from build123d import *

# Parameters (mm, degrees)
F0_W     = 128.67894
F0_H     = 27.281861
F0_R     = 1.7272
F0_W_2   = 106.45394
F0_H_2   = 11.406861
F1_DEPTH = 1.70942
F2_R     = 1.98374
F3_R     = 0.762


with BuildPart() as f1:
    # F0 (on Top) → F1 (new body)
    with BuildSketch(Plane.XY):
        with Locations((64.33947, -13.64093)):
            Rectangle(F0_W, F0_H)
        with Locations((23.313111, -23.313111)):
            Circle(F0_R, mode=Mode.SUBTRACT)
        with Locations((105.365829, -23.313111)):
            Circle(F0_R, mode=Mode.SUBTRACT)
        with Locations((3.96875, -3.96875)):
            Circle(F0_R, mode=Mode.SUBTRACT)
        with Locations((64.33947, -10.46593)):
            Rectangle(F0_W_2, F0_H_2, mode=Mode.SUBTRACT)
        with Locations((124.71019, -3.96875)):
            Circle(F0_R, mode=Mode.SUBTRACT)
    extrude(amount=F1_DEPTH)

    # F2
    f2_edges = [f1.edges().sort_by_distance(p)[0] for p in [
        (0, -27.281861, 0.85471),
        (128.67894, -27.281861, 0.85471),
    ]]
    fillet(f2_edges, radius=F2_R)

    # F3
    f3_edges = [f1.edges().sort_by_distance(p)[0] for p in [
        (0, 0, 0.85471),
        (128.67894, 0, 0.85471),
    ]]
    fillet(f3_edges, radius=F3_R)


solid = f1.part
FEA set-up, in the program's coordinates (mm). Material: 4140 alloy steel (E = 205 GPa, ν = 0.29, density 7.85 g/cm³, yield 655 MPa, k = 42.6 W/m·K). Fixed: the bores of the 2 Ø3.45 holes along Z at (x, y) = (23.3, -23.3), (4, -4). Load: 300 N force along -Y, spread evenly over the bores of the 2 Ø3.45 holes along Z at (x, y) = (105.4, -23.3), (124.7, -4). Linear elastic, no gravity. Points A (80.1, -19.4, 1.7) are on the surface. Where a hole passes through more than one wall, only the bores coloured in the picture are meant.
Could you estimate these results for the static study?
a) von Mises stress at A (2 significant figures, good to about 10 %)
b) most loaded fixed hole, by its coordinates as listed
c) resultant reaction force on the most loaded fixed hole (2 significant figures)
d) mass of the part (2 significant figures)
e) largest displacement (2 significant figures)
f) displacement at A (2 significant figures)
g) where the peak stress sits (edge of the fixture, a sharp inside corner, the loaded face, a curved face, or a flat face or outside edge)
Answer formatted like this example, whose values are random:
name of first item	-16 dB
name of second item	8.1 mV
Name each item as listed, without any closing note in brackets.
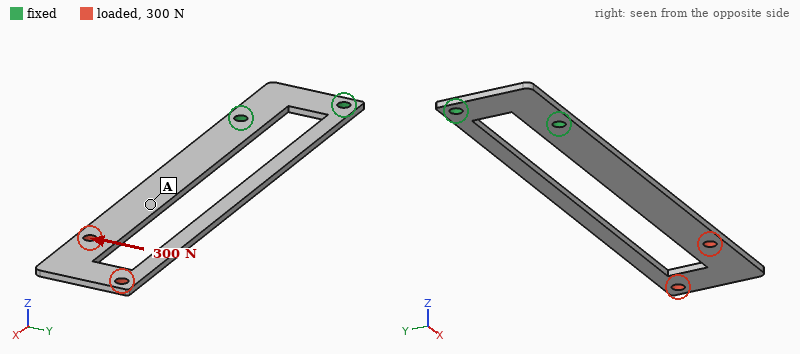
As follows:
von Mises stress at A	56 MPa
most loaded fixed hole, by its coordinates as listed	(23.3, -23.3)
resultant reaction force on the most loaded fixed hole	920 N
mass of the part	30 g
largest displacement	0.84 mm
displacement at A	0.46 mm
where the peak stress sits	edge of the fixture
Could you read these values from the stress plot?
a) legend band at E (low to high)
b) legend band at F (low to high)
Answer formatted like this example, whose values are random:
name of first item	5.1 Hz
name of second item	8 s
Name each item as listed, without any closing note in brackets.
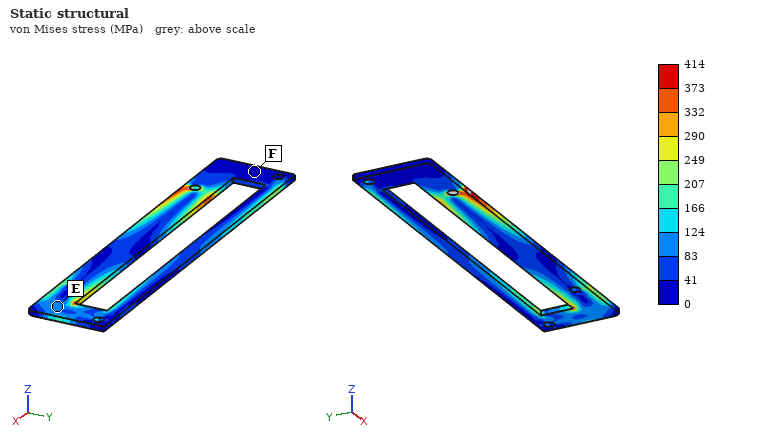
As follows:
legend band at E	83 to 124 MPa
legend band at F	0 to 41 MPa
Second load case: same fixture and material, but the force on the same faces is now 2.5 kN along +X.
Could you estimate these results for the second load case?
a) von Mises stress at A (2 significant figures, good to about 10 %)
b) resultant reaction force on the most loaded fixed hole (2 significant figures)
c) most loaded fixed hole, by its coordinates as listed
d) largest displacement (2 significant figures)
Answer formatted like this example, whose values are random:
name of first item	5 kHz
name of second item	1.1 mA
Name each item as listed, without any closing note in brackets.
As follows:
von Mises stress at A	82 MPa
resultant reaction force on the most loaded fixed hole	1.4 kN
most loaded fixed hole, by its coordinates as listed	(23.3, -23.3)
largest displacement	0.12 mm
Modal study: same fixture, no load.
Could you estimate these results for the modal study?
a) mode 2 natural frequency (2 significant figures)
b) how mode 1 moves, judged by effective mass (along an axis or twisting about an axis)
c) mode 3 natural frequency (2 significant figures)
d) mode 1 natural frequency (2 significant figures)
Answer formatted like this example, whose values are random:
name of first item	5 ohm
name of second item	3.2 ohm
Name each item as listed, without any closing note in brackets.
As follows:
mode 2 natural frequency	550 Hz
how mode 1 moves, judged by effective mass	along Z
mode 3 natural frequency	710 Hz
mode 1 natural frequency	110 Hz
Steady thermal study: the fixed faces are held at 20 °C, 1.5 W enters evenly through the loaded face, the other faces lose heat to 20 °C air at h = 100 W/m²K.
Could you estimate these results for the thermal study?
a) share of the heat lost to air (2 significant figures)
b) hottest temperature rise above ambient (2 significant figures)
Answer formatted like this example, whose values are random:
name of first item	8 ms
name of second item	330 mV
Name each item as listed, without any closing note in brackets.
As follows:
share of the heat lost to air	99 %
hottest temperature rise above ambient	14 K
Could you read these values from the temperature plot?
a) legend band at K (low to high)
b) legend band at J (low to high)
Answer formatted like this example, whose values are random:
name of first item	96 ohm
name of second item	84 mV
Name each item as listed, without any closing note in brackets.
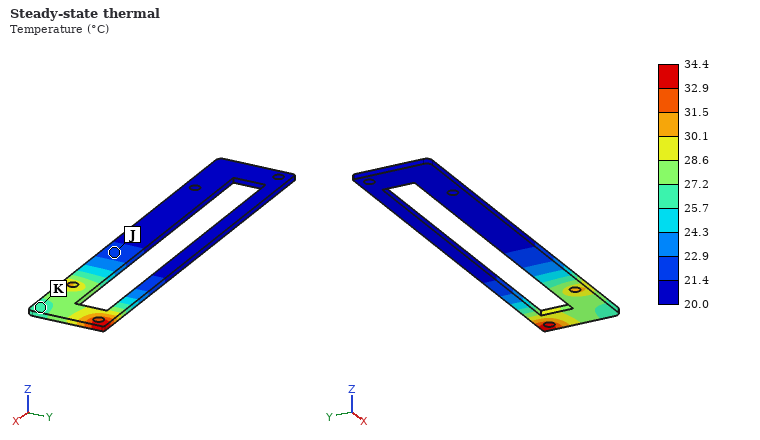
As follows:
legend band at K	25.7 to 27.2 °C
legend band at J	21.4 to 22.9 °C
